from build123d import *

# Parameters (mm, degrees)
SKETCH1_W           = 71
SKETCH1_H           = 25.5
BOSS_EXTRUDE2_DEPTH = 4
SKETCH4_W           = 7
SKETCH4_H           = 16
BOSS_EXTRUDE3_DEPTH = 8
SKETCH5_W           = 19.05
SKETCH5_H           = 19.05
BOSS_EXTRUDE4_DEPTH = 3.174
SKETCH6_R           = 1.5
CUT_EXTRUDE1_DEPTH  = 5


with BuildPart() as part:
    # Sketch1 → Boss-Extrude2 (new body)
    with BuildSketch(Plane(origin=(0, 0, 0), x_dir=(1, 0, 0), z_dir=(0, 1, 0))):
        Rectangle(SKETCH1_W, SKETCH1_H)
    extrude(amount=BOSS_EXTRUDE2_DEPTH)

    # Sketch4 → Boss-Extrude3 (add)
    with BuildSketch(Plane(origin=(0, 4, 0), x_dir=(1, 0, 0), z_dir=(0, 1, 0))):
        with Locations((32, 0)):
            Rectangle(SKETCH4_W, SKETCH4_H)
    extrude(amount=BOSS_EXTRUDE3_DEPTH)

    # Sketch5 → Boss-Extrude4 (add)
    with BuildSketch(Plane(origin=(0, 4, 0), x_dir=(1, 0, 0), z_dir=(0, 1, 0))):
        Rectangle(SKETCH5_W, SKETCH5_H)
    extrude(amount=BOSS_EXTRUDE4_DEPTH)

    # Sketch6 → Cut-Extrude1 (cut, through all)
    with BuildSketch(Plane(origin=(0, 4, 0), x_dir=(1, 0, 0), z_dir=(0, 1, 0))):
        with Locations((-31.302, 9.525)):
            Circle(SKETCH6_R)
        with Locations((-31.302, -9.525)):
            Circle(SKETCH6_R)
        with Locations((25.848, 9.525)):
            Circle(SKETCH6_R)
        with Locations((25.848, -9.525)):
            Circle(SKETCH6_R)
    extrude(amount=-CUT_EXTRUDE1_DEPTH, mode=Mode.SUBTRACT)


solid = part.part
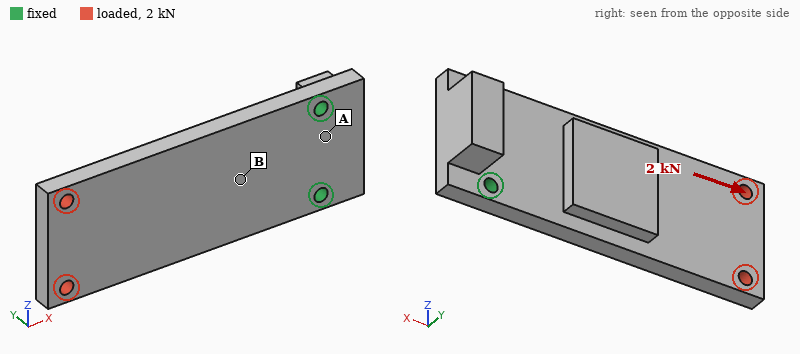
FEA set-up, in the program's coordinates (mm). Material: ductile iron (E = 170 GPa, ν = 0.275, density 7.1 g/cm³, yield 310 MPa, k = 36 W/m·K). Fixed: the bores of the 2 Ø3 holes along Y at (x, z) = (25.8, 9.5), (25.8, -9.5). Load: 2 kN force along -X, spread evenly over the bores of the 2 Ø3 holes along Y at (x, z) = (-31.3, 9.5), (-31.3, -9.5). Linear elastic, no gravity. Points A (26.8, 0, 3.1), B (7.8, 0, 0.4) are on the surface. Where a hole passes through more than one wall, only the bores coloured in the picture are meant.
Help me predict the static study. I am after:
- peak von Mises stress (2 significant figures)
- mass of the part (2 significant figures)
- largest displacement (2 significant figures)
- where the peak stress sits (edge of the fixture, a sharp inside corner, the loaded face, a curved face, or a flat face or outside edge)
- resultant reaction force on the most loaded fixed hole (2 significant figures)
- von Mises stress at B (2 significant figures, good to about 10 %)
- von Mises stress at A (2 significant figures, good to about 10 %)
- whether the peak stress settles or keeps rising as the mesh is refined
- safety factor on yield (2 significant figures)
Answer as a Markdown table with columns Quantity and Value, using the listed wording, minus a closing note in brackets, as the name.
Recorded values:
| Quantity | Value |
|---|---|
| peak von Mises stress | 81 MPa |
| mass of the part | 65 g |
| largest displacement | 16 µm |
| where the peak stress sits | the loaded face |
| resultant reaction force on the most loaded fixed hole | 1.0 kN |
| von Mises stress at B | 22 MPa |
| von Mises stress at A | 8.0 MPa |
| whether the peak stress settles or keeps rising as the mesh is refined | settles |
| safety factor on yield | 3.8 |
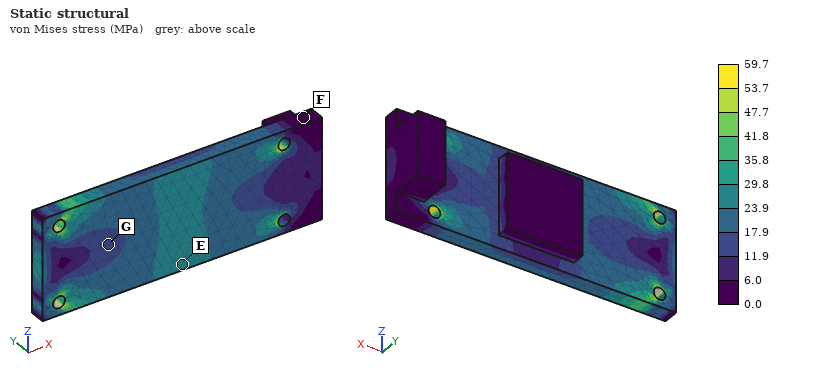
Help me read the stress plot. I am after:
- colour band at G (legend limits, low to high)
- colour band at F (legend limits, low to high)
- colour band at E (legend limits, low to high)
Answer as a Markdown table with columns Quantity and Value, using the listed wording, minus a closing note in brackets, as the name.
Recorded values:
| Quantity | Value |
|---|---|
| colour band at G | 11.9 to 17.9 MPa |
| colour band at F | 0.0 to 6.0 MPa |
| colour band at E | 23.9 to 29.8 MPa |
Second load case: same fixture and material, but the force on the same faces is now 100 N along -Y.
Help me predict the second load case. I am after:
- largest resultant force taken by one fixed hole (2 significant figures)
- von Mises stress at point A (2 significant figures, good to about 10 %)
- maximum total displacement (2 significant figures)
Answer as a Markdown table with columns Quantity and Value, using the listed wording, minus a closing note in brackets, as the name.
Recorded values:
| Quantity | Value |
|---|---|
| largest resultant force taken by one fixed hole | 54 N |
| von Mises stress at point A | 28 MPa |
| maximum total displacement | 0.24 mm |
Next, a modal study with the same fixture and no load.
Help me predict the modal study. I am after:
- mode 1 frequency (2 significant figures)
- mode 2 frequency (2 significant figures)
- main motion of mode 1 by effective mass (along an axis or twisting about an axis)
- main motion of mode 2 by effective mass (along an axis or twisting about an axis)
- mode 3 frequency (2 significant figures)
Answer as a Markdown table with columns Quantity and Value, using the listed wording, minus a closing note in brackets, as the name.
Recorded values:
| Quantity | Value |
|---|---|
| mode 1 frequency | 890 Hz |
| mode 2 frequency | 4800 Hz |
| main motion of mode 1 by effective mass | along Y |
| main motion of mode 2 by effective mass | along Z |
| mode 3 frequency | 5200 Hz |
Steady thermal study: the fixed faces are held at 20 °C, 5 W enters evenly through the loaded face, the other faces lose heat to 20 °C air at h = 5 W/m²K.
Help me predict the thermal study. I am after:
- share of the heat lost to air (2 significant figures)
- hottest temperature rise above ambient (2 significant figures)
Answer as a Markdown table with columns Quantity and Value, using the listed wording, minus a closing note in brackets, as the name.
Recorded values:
| Quantity | Value |
|---|---|
| share of the heat lost to air | 14 % |
| hottest temperature rise above ambient | 70 K |
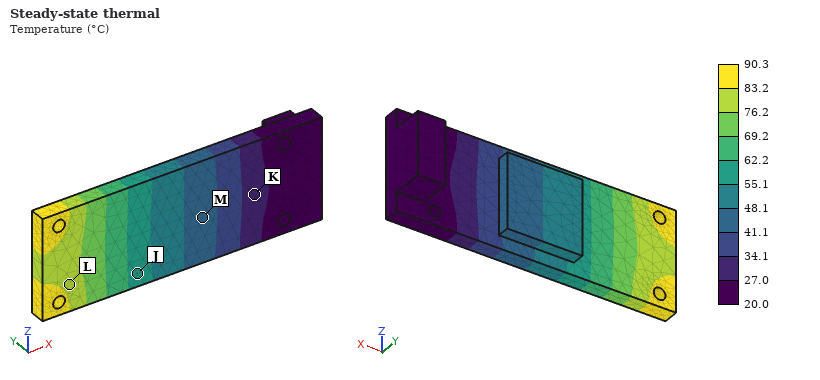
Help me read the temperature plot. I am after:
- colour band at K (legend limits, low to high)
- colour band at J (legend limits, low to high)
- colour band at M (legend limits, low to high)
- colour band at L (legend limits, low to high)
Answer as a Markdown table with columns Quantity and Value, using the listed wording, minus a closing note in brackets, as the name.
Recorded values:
| Quantity | Value |
|---|---|
| colour band at K | 27.0 to 34.1 °C |
| colour band at J | 55.1 to 62.2 °C |
| colour band at M | 41.1 to 48.1 °C |
| colour band at L | 76.2 to 83.2 °C |
